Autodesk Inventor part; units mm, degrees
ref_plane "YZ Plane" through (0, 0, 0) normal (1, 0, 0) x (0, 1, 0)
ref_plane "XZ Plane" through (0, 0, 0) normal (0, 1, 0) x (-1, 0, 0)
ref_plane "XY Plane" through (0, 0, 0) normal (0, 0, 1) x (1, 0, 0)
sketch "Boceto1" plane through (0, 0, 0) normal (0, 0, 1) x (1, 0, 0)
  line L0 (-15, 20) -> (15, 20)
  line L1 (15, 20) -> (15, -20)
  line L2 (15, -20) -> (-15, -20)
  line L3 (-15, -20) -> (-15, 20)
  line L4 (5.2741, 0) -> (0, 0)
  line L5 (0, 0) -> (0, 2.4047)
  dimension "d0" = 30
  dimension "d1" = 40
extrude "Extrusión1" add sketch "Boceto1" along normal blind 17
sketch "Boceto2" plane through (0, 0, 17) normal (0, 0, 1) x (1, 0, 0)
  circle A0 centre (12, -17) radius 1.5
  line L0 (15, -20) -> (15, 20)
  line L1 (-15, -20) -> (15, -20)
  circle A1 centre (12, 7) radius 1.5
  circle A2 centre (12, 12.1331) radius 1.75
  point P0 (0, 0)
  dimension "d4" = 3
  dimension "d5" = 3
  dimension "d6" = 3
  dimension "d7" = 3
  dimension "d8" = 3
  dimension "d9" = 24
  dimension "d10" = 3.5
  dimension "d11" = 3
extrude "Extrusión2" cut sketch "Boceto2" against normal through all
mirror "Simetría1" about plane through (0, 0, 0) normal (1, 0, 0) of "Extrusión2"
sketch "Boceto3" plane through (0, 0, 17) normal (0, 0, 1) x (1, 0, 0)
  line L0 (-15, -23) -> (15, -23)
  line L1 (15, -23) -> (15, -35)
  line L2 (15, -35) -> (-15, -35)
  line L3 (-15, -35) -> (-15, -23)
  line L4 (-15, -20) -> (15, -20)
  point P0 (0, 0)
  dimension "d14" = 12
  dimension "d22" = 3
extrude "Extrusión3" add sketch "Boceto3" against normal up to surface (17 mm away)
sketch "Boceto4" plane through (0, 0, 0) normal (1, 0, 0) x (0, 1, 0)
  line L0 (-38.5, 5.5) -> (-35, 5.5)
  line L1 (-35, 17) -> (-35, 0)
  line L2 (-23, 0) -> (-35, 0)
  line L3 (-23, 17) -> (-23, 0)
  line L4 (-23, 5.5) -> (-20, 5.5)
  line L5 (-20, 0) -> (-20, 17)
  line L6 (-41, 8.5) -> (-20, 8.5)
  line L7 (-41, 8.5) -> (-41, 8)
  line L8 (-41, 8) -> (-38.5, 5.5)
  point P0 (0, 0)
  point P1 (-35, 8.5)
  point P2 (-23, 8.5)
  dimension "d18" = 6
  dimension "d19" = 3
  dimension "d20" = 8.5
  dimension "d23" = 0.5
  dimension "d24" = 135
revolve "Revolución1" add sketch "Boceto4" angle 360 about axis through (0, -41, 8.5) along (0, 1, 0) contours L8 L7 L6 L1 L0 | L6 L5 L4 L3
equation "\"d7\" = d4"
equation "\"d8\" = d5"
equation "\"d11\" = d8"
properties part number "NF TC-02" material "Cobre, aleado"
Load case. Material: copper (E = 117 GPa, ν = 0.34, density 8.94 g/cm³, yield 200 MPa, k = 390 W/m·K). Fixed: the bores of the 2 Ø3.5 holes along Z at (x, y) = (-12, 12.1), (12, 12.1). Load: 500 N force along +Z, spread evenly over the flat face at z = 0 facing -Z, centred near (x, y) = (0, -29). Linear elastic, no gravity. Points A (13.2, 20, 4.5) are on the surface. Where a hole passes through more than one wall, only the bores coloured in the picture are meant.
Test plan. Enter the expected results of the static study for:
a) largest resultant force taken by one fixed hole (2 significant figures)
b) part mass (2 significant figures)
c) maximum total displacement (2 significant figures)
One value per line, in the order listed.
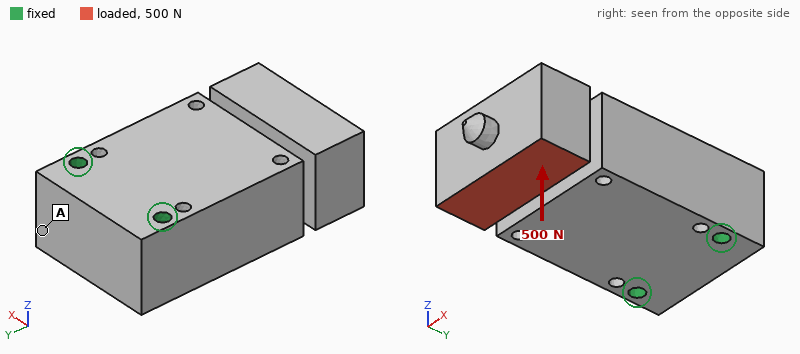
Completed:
250 N
230 g
72 µm
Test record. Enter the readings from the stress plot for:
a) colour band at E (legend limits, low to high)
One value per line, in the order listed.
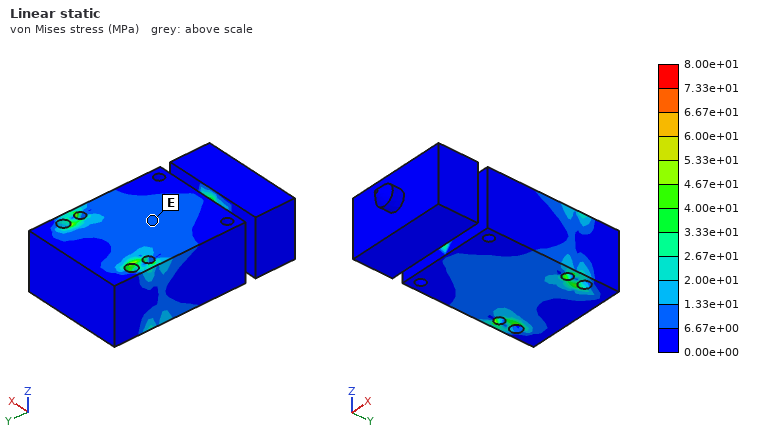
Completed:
6.67e+00 to 1.33e+01 MPa
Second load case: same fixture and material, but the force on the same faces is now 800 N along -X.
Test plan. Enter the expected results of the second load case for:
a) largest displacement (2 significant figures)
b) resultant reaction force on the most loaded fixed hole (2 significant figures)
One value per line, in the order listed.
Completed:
0.16 mm
1.4 kN
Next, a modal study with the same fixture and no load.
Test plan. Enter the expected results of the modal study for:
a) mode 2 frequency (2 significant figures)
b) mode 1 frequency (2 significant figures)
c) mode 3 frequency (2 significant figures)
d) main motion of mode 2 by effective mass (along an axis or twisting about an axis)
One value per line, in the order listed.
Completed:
2200 Hz
2000 Hz
2300 Hz
along Z
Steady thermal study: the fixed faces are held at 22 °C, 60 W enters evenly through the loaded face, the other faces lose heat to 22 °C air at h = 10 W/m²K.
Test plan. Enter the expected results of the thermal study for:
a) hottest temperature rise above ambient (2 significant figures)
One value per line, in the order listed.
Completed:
49 K
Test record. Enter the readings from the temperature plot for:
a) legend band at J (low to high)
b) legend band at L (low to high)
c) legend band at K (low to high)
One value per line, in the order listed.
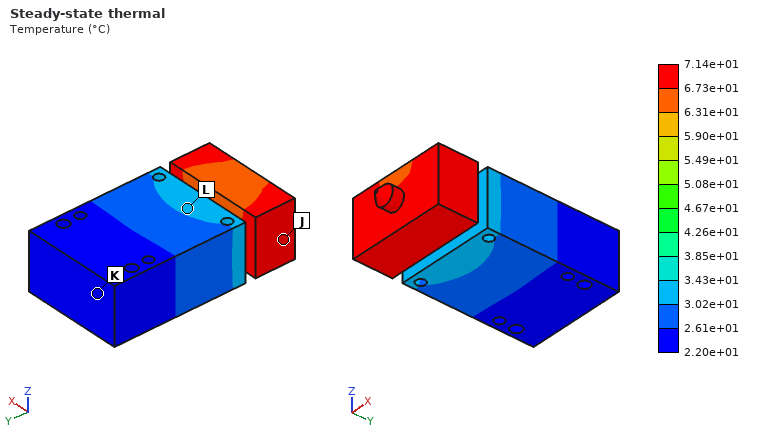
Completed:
6.73e+01 to 7.14e+01 °C
3.02e+01 to 3.43e+01 °C
2.20e+01 to 2.61e+01 °C
